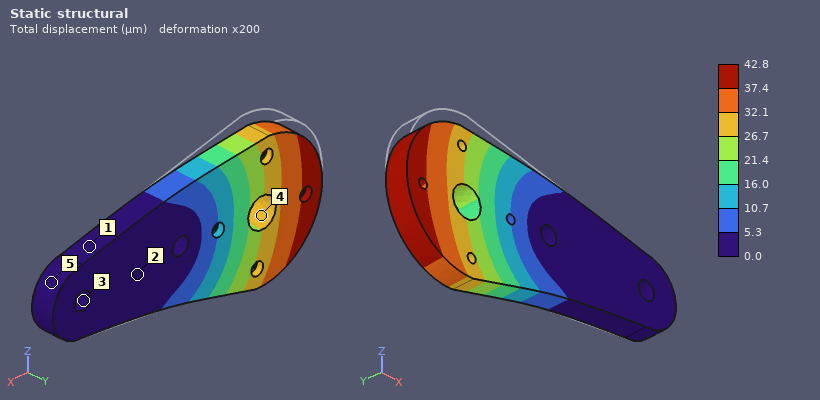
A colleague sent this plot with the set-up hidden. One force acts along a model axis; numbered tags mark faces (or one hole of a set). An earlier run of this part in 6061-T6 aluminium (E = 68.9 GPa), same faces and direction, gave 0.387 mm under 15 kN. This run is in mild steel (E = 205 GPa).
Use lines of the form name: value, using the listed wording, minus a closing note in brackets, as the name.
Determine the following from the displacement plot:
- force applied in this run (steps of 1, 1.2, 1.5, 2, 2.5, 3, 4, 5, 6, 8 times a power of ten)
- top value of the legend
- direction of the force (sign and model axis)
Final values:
force applied in this run: 5 kN
top value of the legend: 42.8 µm
direction of the force: -Z
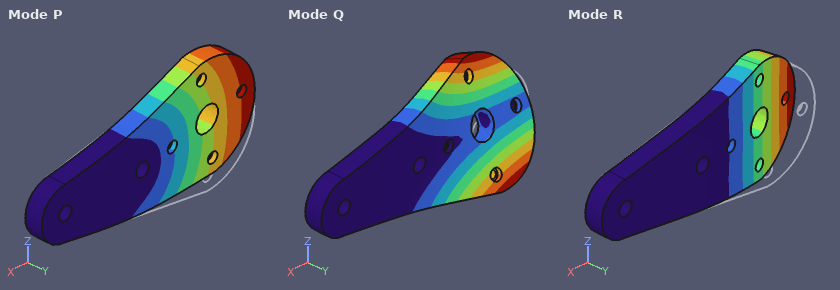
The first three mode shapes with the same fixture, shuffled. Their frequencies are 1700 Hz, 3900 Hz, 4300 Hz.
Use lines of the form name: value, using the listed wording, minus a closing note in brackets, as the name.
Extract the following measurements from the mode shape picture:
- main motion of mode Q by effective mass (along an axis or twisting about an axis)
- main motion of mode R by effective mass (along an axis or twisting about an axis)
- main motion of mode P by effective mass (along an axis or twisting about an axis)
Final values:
main motion of mode Q by effective mass: twisting about X
main motion of mode R by effective mass: along Y
main motion of mode P by effective mass: along Z
